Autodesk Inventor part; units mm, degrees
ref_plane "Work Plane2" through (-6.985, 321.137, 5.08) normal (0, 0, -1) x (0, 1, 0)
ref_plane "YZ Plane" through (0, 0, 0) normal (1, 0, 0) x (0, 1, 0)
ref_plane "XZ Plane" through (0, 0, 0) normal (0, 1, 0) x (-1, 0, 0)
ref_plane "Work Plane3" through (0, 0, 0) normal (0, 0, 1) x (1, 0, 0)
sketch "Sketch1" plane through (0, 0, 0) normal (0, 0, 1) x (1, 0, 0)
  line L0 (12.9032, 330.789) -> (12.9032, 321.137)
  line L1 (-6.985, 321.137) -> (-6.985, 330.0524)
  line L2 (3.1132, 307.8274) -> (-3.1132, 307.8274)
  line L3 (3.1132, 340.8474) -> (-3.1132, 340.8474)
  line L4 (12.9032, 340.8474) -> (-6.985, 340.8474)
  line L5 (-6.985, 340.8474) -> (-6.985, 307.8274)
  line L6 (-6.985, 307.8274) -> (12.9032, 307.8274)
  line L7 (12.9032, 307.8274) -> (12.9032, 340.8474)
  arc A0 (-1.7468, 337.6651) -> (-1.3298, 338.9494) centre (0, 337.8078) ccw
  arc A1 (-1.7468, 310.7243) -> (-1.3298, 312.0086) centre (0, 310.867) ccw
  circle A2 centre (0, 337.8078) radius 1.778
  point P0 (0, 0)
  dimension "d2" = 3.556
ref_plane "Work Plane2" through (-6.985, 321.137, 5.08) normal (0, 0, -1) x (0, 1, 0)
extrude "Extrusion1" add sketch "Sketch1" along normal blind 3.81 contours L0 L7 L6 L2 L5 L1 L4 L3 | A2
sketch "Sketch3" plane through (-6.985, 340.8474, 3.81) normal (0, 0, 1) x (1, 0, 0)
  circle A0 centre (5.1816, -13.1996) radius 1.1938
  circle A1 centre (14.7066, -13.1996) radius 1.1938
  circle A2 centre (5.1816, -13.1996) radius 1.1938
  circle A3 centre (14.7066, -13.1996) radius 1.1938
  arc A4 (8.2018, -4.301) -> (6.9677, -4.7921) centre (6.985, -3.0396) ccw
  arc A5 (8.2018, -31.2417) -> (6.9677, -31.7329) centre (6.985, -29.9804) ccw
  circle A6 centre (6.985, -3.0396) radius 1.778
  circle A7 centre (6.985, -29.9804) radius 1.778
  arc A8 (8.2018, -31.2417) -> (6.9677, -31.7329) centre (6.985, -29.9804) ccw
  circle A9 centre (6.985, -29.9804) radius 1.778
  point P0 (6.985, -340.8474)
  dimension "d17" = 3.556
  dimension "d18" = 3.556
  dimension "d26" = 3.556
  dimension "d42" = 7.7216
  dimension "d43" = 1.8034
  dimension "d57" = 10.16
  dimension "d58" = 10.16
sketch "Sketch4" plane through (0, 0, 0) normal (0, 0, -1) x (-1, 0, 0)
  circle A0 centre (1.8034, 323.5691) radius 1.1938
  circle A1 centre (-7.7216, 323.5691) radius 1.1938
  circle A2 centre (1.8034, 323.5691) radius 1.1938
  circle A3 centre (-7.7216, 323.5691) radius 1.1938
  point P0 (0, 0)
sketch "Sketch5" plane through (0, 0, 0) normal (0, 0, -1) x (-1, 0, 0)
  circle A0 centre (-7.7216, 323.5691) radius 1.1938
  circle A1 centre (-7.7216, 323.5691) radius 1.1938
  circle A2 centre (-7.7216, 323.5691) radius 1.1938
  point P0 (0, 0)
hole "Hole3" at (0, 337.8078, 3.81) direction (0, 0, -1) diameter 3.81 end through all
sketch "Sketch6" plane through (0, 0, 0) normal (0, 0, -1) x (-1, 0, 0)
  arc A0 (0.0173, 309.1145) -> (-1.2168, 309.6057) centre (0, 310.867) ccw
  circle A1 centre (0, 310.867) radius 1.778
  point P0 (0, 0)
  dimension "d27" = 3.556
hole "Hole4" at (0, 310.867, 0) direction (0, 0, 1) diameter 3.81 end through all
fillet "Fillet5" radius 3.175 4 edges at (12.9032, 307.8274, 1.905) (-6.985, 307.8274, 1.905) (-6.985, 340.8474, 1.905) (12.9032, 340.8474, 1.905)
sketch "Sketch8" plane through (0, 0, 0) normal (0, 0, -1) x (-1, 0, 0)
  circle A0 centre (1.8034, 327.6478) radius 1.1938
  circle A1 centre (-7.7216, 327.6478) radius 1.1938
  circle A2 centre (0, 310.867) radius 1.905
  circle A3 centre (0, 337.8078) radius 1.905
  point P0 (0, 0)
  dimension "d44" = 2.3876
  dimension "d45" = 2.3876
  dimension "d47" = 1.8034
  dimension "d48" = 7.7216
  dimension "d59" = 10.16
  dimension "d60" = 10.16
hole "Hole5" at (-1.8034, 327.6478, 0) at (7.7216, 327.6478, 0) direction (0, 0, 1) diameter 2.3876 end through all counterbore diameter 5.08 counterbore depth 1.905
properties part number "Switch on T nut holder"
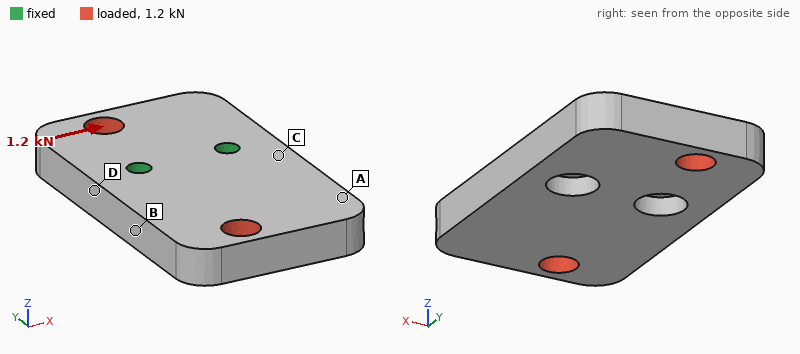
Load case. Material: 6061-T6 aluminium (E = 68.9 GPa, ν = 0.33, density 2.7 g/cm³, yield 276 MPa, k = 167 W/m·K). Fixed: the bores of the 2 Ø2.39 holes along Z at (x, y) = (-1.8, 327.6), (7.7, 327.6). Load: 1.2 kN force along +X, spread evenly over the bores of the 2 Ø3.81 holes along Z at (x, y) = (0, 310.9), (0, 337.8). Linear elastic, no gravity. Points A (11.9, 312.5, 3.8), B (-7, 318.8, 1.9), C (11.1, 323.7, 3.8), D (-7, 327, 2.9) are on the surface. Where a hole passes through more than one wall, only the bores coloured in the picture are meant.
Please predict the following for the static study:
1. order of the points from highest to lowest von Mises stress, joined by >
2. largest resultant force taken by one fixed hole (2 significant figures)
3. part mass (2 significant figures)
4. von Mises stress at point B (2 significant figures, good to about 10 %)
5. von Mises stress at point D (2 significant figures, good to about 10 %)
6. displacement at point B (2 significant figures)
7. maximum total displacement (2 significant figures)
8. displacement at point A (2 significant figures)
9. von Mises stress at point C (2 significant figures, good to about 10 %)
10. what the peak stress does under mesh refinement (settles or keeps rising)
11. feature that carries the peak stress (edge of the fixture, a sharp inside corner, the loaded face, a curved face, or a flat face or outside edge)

D > C > B > A
720 N
6.2 g
21 MPa
46 MPa
10 µm
20 µm
15 µm
28 MPa
keeps rising
edge of the fixture
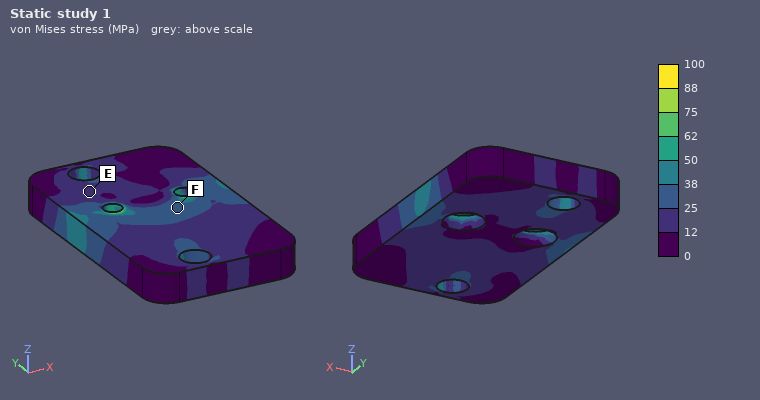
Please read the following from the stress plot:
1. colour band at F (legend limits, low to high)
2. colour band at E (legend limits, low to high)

25 to 38 MPa
12 to 25 MPa
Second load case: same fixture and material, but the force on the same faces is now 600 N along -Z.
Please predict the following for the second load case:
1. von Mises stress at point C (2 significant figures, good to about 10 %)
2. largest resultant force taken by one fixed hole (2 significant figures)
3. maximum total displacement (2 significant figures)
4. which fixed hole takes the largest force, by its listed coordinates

75 MPa
470 N
0.16 mm
(-1.8, 327.6)
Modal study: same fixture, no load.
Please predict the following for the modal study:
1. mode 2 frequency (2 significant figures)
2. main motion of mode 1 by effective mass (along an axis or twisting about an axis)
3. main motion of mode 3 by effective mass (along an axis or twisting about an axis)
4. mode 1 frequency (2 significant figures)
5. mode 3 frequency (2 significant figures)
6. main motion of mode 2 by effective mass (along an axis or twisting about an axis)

13 kHz
along Z
twisting about Y
5400 Hz
15 kHz
along Z
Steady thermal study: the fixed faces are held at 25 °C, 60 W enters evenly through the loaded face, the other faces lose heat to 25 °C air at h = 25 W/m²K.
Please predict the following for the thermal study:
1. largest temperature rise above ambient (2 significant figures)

65 K
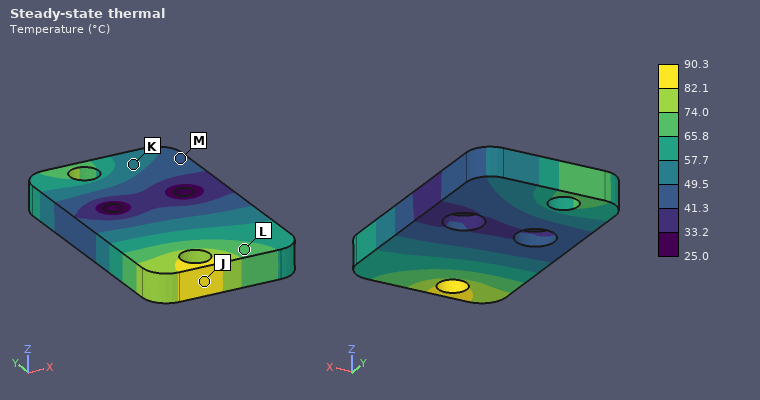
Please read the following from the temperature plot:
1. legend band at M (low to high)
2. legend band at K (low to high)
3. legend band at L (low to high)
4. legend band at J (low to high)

41.3 to 49.5 °C
49.5 to 57.7 °C
65.8 to 74.0 °C
82.1 to 90.3 °C
